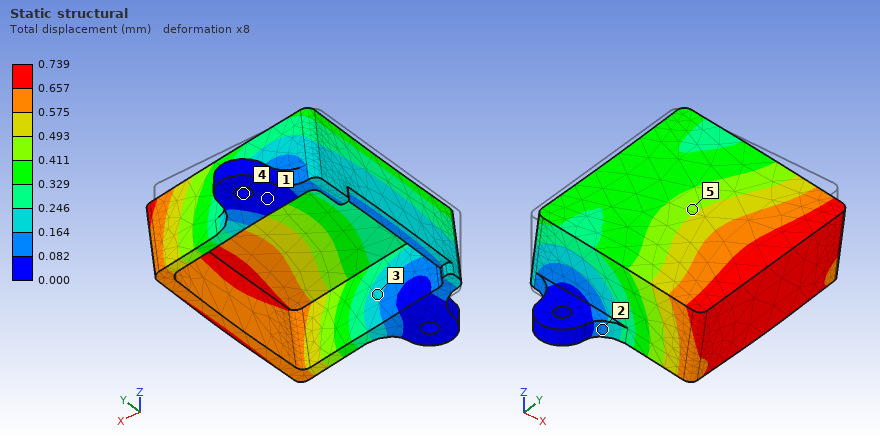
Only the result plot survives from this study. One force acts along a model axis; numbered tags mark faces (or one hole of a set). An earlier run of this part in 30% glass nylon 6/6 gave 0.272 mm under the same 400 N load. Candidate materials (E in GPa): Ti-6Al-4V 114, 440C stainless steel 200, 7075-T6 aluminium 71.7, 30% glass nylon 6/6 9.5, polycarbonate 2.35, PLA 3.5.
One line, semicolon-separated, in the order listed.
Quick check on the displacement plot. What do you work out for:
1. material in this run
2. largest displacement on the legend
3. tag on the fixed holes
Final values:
PLA; 0.739 mm; 4
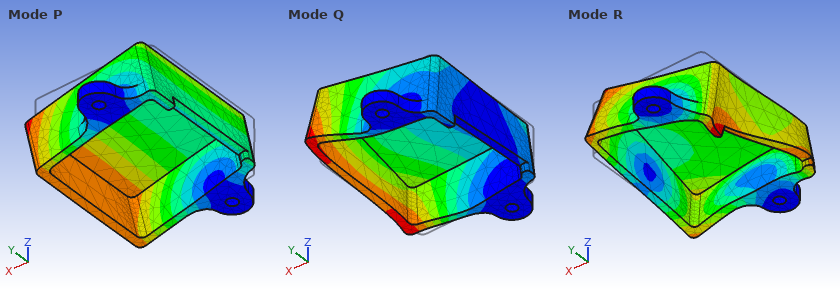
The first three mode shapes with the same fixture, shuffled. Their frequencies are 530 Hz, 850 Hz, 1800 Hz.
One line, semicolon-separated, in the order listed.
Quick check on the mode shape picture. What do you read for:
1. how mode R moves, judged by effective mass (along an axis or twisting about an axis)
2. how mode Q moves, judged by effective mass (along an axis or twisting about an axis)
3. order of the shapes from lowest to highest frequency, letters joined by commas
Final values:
along Y; along Y; P, Q, R
